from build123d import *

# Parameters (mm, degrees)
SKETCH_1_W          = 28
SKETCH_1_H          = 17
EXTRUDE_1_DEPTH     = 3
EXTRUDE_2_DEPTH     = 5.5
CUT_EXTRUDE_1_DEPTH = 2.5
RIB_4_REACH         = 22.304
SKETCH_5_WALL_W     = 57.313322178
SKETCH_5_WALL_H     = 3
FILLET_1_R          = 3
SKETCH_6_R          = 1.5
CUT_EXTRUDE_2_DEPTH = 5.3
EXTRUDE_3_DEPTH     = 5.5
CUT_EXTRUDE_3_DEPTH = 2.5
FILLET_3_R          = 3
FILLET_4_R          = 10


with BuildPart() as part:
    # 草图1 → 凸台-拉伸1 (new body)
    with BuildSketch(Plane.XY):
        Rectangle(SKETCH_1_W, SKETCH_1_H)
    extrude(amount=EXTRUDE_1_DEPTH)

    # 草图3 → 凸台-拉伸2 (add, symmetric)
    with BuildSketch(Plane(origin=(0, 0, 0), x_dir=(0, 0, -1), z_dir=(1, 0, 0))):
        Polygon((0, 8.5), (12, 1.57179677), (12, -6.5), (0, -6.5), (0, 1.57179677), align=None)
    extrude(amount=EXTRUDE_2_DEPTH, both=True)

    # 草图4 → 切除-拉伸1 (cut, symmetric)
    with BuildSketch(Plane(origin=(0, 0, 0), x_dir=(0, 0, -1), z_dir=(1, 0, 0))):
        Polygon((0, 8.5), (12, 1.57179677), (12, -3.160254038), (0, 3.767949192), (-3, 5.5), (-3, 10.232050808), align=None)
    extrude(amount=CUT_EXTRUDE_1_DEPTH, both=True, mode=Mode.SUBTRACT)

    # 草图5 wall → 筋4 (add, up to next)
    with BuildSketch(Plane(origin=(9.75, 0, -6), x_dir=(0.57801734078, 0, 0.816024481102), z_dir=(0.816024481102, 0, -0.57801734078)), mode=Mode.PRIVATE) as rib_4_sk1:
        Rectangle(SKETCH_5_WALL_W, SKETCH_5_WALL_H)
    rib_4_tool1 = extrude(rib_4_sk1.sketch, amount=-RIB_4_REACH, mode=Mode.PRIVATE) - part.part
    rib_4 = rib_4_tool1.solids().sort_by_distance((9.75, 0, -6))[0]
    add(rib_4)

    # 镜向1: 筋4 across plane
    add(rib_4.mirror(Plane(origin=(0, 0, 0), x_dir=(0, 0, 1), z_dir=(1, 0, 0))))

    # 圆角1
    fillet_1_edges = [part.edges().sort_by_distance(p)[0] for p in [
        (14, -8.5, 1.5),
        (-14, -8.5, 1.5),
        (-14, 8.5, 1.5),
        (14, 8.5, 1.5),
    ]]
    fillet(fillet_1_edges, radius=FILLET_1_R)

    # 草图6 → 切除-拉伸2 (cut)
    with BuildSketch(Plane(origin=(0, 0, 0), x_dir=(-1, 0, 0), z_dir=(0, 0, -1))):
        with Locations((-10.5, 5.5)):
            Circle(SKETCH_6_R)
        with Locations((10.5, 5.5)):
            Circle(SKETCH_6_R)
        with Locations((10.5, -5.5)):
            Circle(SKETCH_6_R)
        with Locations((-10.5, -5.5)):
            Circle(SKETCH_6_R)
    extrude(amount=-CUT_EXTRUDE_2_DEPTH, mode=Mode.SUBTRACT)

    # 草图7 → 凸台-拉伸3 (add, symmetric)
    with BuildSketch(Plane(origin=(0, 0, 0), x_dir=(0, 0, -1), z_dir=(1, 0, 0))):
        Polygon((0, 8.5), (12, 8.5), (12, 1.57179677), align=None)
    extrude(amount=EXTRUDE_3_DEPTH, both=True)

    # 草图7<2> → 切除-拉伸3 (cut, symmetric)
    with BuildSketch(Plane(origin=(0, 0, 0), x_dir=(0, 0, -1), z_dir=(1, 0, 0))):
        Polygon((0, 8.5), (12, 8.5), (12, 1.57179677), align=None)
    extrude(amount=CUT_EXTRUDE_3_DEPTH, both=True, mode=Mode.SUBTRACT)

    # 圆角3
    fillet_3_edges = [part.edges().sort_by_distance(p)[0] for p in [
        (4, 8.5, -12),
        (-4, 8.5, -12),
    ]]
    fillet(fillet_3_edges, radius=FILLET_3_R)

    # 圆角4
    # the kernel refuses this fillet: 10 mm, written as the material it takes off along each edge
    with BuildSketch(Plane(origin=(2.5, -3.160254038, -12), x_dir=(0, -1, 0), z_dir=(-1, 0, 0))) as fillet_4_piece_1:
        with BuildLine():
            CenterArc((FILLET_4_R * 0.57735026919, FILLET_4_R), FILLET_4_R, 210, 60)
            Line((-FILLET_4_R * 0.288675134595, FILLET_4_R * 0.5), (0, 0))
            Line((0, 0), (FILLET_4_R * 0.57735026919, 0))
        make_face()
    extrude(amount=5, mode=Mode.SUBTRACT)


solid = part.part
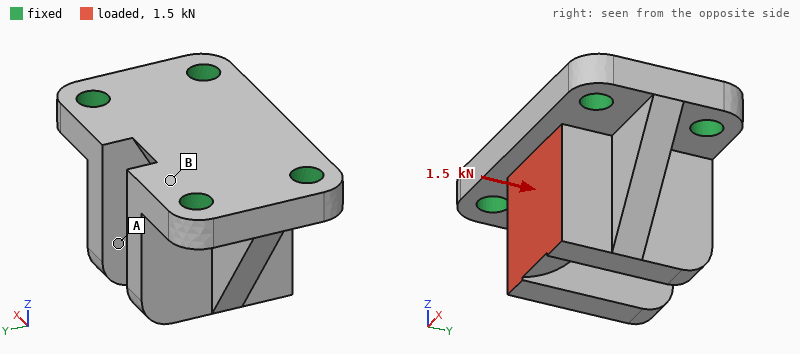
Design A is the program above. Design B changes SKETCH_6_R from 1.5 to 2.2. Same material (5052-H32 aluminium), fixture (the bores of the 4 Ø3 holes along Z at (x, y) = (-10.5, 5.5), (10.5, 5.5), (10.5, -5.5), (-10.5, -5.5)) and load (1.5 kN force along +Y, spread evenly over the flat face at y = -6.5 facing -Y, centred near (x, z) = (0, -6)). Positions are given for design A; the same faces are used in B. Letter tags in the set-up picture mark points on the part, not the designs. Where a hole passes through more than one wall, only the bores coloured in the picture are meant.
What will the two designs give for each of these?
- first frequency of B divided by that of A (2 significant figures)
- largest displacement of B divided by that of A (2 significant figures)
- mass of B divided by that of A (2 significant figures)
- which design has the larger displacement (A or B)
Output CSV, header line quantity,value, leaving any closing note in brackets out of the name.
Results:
quantity,value
first frequency of B divided by that of A,1.1
largest displacement of B divided by that of A,0.81
mass of B divided by that of A,0.97
which design has the larger displacement,A
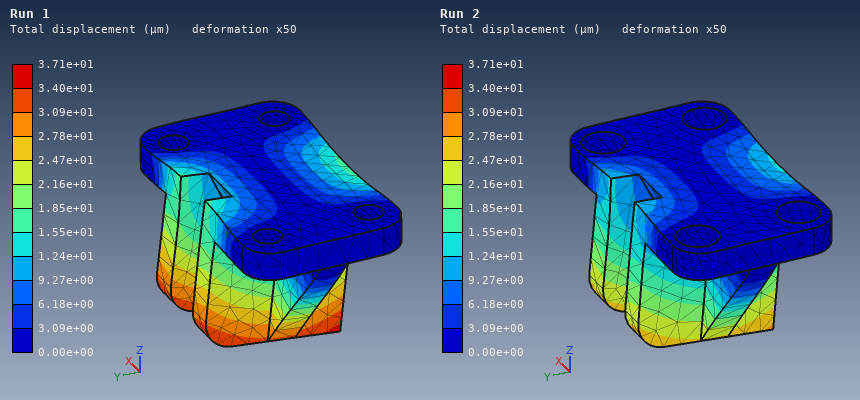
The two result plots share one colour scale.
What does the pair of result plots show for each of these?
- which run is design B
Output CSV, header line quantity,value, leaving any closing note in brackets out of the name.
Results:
quantity,value
which run is design B,Run 2
